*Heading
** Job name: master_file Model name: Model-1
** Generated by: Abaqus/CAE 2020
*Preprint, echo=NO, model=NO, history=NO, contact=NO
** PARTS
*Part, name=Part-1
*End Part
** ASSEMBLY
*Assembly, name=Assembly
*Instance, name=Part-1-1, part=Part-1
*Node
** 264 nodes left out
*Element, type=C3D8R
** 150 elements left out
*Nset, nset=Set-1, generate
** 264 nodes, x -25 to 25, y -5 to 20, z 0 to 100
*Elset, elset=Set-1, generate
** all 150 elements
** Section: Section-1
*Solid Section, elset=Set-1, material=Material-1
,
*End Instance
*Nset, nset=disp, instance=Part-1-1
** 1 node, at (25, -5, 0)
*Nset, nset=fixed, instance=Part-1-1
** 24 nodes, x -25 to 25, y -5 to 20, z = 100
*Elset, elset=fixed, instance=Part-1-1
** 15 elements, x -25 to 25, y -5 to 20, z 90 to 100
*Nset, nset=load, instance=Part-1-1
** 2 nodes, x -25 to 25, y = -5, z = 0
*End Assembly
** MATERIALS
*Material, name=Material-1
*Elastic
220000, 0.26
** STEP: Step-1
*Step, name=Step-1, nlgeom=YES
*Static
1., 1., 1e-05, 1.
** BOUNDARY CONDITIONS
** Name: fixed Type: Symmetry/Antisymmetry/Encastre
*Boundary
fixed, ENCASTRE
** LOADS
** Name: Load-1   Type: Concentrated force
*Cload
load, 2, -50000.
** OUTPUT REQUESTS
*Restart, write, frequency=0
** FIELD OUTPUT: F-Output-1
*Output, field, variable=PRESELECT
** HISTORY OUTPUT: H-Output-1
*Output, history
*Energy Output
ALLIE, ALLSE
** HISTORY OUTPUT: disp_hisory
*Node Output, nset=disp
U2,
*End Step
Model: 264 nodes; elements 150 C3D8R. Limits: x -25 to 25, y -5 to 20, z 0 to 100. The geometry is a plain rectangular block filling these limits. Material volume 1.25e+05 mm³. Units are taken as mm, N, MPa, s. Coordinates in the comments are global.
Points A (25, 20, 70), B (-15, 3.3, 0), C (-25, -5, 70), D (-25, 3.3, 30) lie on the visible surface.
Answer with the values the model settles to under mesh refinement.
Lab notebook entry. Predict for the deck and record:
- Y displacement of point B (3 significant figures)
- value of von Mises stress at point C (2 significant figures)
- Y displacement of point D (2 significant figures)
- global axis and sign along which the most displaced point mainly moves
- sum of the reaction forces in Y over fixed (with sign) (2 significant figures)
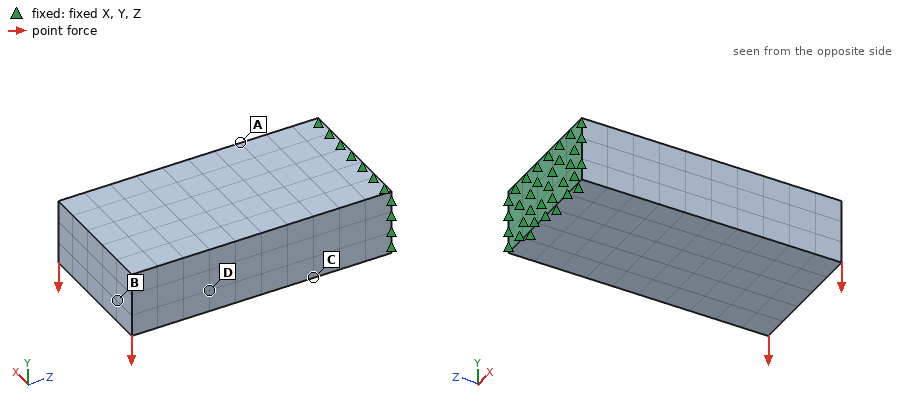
-2.35 mm
1300 MPa
-1.3 mm
-Y
1.0e+05 N
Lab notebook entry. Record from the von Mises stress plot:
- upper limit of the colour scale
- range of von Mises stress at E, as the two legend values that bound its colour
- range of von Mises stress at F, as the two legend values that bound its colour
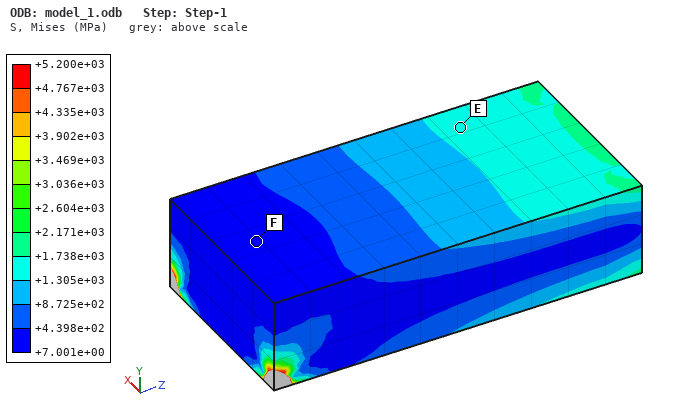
+5.200e+03 MPa
+1.305e+03 to +1.738e+03 MPa
+7.001e+00 to +4.398e+02 MPa
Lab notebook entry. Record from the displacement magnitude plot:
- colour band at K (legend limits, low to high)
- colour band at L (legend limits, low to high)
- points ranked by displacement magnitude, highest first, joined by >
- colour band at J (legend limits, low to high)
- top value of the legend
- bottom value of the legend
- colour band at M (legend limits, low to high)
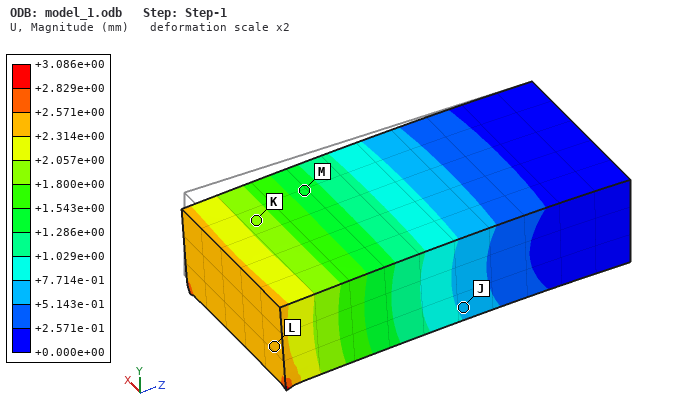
+1.800e+00 to +2.057e+00 mm
+2.314e+00 to +2.571e+00 mm
L > K > M > J
+5.143e-01 to +7.714e-01 mm
+3.086e+00 mm
+0.000e+00 mm
+1.286e+00 to +1.543e+00 mm
